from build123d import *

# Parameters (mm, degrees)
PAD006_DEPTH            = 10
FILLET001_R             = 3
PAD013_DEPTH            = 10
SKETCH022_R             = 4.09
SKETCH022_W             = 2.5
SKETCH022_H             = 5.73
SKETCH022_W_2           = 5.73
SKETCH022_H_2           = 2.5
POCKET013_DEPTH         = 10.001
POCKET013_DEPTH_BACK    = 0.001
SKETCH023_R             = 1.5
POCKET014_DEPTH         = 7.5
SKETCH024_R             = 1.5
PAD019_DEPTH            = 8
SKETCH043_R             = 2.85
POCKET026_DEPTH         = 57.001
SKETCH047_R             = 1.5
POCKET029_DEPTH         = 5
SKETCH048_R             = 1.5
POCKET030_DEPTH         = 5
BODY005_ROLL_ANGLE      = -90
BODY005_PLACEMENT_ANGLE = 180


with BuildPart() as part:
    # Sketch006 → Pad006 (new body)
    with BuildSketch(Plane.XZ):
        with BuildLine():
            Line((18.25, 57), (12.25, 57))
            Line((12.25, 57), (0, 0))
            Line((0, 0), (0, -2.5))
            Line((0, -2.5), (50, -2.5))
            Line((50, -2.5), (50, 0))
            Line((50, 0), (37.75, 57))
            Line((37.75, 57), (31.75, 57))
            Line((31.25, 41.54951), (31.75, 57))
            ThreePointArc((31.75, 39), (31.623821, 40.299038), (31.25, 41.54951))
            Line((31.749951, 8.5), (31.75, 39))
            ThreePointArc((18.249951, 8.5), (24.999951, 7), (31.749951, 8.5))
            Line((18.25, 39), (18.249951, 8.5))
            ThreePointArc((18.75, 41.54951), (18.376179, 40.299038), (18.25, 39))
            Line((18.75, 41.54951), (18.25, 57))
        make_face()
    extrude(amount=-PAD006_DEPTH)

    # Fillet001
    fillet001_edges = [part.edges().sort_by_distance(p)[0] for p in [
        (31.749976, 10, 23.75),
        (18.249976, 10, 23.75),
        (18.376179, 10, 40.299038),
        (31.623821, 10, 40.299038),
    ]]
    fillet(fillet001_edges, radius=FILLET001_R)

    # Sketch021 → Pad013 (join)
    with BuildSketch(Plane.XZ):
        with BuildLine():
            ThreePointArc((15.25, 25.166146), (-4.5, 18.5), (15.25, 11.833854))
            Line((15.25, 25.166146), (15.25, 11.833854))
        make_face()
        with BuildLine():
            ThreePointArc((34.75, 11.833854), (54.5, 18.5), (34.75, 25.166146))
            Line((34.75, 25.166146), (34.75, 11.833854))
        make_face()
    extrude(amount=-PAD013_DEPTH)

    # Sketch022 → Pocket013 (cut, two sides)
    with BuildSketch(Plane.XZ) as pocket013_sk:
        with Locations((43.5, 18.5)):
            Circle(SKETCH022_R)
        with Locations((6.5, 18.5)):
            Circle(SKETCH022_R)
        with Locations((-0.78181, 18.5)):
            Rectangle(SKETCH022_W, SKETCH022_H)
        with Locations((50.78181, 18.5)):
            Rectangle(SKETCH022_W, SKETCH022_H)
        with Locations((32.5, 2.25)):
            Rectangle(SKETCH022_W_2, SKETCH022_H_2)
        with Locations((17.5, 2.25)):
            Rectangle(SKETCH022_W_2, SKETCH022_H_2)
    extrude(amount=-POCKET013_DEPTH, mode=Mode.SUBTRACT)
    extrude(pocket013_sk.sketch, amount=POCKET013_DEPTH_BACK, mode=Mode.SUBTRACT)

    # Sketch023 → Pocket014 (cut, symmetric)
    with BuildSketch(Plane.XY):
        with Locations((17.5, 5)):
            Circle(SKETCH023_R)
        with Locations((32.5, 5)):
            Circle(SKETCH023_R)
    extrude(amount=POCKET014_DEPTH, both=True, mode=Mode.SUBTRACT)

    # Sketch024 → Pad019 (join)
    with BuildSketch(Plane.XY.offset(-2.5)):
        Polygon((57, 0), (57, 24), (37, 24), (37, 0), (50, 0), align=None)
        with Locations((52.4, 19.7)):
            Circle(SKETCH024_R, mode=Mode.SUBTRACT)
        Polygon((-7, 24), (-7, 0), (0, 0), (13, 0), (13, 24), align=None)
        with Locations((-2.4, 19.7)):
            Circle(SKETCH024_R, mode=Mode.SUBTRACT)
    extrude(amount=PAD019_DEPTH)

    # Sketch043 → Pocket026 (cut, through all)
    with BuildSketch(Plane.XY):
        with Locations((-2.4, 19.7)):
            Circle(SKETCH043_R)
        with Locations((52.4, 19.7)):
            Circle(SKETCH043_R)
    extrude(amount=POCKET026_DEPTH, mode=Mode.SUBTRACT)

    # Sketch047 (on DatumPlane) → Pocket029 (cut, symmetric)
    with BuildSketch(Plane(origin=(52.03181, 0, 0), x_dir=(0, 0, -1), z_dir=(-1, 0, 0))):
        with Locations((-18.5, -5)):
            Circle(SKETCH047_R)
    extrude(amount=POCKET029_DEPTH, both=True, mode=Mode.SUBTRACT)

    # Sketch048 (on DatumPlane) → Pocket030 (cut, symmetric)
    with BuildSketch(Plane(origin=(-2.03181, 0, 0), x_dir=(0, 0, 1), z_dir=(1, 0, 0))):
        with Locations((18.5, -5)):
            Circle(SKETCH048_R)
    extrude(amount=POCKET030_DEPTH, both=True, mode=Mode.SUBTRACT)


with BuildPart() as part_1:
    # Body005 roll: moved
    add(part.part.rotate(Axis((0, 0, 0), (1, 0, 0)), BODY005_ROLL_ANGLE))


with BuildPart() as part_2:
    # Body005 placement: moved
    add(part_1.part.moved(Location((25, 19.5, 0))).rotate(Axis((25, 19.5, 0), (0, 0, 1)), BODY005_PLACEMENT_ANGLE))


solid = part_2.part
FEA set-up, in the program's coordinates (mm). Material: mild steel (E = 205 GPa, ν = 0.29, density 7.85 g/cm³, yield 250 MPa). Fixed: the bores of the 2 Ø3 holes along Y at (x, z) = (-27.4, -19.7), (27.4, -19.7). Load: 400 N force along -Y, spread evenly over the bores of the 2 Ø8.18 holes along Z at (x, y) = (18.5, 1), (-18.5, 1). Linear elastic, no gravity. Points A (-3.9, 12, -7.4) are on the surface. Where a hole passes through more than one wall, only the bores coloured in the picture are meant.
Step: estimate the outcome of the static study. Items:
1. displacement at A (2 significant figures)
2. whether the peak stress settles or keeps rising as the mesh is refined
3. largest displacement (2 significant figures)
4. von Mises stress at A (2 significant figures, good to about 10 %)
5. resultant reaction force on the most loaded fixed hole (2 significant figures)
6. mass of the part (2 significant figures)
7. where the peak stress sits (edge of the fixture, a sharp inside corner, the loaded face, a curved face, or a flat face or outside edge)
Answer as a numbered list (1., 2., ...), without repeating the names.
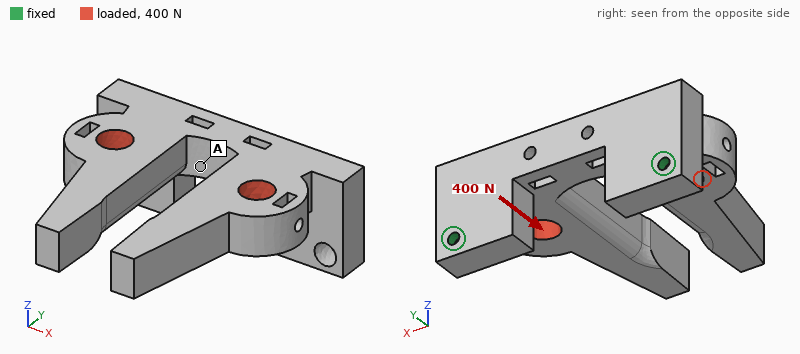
1. 16 µm
2. keeps rising
3. 61 µm
4. 12 MPa
5. 200 N
6. 180 g
7. edge of the fixture
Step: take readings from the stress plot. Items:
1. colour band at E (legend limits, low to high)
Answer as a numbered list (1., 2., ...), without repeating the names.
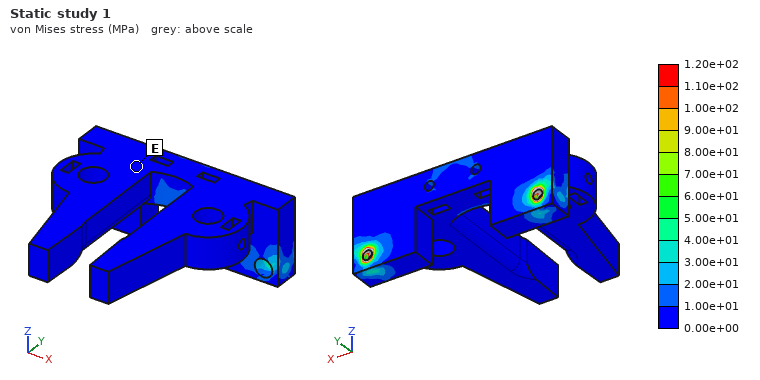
1. 0.00e+00 to 1.00e+01 MPa
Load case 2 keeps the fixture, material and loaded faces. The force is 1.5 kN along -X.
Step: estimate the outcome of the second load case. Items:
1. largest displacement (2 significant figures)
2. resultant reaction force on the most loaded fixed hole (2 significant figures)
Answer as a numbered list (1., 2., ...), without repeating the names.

1. 48 µm
2. 980 N
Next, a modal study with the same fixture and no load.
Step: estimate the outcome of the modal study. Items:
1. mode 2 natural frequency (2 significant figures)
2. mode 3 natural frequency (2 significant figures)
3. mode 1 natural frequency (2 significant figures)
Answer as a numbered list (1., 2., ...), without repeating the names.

1. 1900 Hz
2. 2600 Hz
3. 990 Hz
